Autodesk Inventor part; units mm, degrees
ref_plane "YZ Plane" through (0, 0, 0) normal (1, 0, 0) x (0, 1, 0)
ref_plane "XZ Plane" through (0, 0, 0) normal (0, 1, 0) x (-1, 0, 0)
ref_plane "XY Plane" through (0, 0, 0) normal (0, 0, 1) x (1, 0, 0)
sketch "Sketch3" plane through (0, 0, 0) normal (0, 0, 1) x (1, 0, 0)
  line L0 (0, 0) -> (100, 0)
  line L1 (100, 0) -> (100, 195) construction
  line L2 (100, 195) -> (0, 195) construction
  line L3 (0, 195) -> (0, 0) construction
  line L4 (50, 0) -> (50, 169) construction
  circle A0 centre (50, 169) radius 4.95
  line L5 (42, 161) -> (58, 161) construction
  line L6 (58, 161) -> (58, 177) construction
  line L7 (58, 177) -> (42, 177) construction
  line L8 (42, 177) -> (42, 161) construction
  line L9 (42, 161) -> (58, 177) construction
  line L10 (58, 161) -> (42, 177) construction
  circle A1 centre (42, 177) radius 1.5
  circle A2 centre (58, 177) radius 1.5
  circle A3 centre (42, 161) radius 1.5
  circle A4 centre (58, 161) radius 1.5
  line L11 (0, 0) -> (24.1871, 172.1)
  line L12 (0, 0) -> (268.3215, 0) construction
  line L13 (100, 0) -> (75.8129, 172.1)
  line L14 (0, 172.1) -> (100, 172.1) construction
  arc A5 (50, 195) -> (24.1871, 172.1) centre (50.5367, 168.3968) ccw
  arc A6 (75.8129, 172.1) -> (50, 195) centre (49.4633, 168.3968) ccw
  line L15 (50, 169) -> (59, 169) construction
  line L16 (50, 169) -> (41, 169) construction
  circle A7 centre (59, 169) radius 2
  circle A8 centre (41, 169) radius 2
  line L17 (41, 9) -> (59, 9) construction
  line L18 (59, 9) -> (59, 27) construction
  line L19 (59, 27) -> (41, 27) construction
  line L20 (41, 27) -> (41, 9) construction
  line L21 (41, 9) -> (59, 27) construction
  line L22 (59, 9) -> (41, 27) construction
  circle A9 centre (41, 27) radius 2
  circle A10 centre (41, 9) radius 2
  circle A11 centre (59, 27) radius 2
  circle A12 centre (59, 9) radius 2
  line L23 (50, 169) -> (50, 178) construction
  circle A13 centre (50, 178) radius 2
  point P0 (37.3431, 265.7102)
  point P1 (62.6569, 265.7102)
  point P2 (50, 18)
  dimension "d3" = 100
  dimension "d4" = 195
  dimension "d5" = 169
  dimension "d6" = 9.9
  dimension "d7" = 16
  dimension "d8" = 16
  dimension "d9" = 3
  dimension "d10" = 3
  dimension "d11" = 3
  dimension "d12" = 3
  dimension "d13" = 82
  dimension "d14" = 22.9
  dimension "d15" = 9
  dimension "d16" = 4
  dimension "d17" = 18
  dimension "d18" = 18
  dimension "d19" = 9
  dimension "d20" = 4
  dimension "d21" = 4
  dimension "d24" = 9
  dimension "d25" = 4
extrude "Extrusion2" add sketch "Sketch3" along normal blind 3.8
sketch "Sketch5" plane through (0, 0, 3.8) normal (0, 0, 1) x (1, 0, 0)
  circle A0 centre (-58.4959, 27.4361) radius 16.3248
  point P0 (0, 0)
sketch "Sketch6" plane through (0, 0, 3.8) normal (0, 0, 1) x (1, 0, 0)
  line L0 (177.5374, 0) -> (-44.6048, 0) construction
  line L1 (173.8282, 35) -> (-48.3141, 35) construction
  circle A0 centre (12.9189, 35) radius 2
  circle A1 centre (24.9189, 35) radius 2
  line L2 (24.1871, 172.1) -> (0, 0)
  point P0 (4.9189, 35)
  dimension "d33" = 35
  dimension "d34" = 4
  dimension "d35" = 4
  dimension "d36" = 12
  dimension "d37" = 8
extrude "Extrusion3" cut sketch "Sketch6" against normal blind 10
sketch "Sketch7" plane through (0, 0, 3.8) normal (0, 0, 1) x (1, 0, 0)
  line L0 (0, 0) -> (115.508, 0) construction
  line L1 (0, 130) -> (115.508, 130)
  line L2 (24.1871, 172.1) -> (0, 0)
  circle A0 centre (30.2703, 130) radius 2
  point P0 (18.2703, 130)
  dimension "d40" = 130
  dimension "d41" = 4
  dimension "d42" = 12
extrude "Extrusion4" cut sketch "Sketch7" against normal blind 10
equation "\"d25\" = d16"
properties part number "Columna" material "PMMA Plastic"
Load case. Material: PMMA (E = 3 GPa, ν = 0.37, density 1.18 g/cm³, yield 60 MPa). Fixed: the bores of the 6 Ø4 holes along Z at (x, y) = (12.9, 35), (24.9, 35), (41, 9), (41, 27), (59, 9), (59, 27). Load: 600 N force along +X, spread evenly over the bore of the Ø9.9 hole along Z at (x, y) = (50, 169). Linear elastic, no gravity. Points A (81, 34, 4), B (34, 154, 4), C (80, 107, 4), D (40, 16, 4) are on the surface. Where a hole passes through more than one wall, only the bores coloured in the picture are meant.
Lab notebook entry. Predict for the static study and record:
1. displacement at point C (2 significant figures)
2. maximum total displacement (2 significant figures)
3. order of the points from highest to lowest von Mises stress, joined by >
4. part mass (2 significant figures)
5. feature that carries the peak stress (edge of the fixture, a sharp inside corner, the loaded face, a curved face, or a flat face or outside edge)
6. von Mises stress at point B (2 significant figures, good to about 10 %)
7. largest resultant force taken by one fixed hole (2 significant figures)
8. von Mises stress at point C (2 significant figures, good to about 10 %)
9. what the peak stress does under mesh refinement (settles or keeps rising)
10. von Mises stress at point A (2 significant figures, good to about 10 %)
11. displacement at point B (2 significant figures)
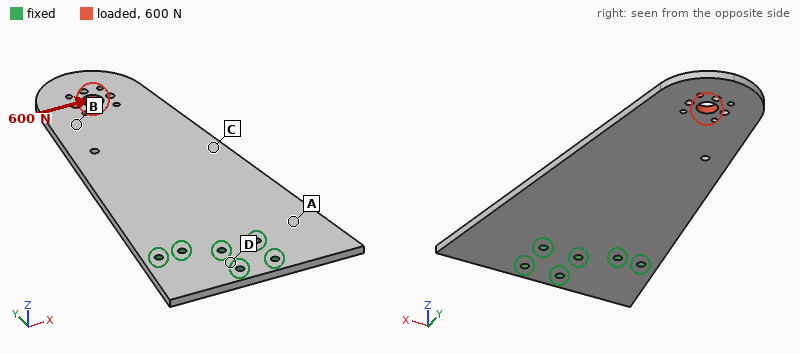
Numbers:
0.86 mm
2.2 mm
C > A > B > D
61 g
edge of the fixture
4.9 MPa
1.1 kN
11 MPa
keeps rising
7.8 MPa
1.5 mm
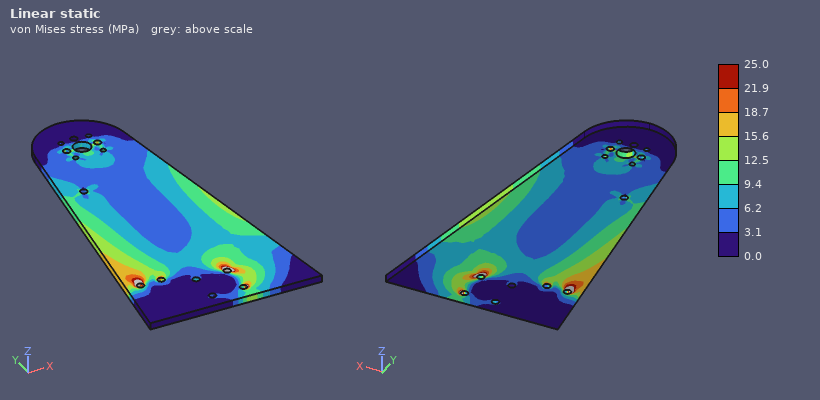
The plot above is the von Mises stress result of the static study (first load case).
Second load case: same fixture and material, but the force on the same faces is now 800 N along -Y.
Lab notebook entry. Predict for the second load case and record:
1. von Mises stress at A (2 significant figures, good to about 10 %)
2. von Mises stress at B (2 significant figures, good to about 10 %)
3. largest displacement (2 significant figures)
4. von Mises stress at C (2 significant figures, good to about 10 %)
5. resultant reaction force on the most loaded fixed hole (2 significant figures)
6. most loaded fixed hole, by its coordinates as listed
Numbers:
1.6 MPa
3.7 MPa
0.24 mm
3.0 MPa
350 N
(59, 27)
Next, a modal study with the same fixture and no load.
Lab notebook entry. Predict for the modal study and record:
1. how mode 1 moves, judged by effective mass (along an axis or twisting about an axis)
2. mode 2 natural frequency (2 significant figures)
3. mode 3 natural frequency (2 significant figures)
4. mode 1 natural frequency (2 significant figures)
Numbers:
along Z
230 Hz
270 Hz
48 Hz
